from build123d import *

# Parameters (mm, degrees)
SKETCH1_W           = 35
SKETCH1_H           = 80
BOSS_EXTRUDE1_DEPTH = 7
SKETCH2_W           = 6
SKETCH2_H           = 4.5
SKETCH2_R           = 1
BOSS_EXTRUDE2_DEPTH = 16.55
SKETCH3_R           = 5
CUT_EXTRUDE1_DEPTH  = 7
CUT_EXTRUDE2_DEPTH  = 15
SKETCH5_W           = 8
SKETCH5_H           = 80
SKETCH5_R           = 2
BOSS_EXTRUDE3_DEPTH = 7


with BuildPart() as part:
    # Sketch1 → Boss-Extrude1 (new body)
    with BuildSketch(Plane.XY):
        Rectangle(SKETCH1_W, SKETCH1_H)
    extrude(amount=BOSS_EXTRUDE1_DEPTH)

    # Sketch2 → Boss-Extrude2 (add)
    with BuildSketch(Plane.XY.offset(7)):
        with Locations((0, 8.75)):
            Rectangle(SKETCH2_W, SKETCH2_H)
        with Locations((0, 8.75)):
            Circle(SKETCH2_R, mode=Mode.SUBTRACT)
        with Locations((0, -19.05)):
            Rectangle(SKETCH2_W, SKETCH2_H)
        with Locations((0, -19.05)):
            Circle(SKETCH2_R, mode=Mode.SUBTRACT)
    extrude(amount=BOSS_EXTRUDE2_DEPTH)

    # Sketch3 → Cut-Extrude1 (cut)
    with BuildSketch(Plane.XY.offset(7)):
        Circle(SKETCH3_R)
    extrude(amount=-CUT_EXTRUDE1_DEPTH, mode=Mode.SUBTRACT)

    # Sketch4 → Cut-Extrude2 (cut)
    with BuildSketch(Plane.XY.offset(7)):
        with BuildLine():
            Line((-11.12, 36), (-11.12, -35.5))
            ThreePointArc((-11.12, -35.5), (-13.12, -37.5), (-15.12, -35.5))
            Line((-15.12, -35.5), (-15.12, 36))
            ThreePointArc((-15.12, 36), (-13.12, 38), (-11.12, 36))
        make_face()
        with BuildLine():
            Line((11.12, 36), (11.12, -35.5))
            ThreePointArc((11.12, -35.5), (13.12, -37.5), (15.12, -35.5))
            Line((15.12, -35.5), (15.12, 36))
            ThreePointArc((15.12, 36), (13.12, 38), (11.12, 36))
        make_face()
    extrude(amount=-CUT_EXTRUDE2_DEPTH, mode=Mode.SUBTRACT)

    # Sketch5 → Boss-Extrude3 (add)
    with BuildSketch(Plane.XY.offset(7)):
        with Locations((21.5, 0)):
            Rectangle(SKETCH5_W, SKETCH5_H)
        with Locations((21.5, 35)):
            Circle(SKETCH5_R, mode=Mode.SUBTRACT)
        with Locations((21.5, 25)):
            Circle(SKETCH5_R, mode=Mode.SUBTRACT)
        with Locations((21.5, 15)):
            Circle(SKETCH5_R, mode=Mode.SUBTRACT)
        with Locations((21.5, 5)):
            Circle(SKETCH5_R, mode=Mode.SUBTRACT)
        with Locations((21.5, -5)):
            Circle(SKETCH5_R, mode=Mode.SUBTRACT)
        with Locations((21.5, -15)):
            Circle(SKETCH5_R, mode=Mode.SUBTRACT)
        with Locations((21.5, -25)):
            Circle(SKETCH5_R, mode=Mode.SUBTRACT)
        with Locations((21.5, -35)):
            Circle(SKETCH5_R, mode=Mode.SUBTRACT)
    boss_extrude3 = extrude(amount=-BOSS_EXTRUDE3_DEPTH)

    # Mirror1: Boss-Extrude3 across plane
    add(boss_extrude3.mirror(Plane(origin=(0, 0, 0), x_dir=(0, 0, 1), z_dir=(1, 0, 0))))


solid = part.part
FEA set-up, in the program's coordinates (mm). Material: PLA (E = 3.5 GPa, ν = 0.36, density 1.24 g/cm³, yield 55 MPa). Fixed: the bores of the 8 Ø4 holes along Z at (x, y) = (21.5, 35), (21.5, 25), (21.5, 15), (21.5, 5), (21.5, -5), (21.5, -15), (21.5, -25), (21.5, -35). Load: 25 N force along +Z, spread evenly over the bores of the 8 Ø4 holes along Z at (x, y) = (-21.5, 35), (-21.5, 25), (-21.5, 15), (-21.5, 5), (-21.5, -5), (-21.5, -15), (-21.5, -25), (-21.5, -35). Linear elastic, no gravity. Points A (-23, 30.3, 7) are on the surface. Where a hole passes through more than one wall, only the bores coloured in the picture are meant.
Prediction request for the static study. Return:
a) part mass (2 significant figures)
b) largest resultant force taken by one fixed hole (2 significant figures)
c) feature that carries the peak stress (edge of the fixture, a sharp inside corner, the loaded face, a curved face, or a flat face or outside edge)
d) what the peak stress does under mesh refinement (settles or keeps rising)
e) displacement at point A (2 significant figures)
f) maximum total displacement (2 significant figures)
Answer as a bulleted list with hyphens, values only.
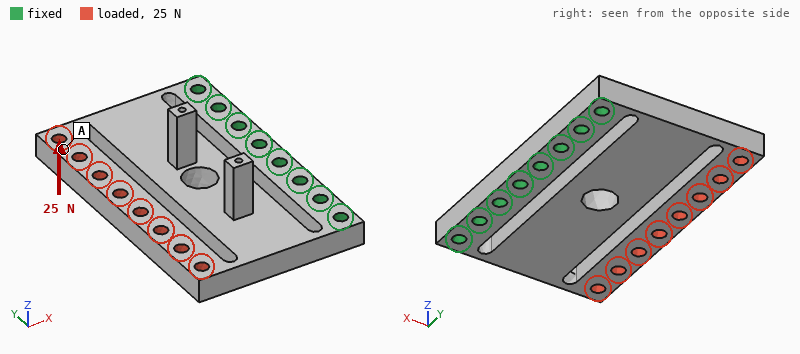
- 29 g
- 11 N
- a sharp inside corner
- keeps rising
- 0.86 mm
- 1.0 mm
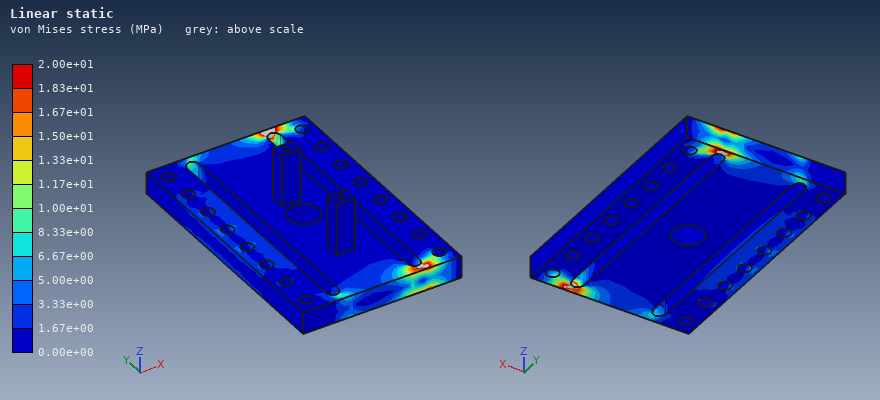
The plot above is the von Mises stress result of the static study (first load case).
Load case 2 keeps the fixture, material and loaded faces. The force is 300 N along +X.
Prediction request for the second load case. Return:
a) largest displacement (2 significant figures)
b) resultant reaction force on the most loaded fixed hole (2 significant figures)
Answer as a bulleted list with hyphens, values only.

- 0.65 mm
- 160 N
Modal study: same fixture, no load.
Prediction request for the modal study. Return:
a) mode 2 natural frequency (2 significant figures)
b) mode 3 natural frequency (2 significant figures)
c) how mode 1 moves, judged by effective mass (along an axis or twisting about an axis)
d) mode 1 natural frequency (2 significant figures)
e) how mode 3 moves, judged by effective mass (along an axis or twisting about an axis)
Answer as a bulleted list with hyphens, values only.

- 920 Hz
- 1000 Hz
- along Z
- 300 Hz
- twisting about X
